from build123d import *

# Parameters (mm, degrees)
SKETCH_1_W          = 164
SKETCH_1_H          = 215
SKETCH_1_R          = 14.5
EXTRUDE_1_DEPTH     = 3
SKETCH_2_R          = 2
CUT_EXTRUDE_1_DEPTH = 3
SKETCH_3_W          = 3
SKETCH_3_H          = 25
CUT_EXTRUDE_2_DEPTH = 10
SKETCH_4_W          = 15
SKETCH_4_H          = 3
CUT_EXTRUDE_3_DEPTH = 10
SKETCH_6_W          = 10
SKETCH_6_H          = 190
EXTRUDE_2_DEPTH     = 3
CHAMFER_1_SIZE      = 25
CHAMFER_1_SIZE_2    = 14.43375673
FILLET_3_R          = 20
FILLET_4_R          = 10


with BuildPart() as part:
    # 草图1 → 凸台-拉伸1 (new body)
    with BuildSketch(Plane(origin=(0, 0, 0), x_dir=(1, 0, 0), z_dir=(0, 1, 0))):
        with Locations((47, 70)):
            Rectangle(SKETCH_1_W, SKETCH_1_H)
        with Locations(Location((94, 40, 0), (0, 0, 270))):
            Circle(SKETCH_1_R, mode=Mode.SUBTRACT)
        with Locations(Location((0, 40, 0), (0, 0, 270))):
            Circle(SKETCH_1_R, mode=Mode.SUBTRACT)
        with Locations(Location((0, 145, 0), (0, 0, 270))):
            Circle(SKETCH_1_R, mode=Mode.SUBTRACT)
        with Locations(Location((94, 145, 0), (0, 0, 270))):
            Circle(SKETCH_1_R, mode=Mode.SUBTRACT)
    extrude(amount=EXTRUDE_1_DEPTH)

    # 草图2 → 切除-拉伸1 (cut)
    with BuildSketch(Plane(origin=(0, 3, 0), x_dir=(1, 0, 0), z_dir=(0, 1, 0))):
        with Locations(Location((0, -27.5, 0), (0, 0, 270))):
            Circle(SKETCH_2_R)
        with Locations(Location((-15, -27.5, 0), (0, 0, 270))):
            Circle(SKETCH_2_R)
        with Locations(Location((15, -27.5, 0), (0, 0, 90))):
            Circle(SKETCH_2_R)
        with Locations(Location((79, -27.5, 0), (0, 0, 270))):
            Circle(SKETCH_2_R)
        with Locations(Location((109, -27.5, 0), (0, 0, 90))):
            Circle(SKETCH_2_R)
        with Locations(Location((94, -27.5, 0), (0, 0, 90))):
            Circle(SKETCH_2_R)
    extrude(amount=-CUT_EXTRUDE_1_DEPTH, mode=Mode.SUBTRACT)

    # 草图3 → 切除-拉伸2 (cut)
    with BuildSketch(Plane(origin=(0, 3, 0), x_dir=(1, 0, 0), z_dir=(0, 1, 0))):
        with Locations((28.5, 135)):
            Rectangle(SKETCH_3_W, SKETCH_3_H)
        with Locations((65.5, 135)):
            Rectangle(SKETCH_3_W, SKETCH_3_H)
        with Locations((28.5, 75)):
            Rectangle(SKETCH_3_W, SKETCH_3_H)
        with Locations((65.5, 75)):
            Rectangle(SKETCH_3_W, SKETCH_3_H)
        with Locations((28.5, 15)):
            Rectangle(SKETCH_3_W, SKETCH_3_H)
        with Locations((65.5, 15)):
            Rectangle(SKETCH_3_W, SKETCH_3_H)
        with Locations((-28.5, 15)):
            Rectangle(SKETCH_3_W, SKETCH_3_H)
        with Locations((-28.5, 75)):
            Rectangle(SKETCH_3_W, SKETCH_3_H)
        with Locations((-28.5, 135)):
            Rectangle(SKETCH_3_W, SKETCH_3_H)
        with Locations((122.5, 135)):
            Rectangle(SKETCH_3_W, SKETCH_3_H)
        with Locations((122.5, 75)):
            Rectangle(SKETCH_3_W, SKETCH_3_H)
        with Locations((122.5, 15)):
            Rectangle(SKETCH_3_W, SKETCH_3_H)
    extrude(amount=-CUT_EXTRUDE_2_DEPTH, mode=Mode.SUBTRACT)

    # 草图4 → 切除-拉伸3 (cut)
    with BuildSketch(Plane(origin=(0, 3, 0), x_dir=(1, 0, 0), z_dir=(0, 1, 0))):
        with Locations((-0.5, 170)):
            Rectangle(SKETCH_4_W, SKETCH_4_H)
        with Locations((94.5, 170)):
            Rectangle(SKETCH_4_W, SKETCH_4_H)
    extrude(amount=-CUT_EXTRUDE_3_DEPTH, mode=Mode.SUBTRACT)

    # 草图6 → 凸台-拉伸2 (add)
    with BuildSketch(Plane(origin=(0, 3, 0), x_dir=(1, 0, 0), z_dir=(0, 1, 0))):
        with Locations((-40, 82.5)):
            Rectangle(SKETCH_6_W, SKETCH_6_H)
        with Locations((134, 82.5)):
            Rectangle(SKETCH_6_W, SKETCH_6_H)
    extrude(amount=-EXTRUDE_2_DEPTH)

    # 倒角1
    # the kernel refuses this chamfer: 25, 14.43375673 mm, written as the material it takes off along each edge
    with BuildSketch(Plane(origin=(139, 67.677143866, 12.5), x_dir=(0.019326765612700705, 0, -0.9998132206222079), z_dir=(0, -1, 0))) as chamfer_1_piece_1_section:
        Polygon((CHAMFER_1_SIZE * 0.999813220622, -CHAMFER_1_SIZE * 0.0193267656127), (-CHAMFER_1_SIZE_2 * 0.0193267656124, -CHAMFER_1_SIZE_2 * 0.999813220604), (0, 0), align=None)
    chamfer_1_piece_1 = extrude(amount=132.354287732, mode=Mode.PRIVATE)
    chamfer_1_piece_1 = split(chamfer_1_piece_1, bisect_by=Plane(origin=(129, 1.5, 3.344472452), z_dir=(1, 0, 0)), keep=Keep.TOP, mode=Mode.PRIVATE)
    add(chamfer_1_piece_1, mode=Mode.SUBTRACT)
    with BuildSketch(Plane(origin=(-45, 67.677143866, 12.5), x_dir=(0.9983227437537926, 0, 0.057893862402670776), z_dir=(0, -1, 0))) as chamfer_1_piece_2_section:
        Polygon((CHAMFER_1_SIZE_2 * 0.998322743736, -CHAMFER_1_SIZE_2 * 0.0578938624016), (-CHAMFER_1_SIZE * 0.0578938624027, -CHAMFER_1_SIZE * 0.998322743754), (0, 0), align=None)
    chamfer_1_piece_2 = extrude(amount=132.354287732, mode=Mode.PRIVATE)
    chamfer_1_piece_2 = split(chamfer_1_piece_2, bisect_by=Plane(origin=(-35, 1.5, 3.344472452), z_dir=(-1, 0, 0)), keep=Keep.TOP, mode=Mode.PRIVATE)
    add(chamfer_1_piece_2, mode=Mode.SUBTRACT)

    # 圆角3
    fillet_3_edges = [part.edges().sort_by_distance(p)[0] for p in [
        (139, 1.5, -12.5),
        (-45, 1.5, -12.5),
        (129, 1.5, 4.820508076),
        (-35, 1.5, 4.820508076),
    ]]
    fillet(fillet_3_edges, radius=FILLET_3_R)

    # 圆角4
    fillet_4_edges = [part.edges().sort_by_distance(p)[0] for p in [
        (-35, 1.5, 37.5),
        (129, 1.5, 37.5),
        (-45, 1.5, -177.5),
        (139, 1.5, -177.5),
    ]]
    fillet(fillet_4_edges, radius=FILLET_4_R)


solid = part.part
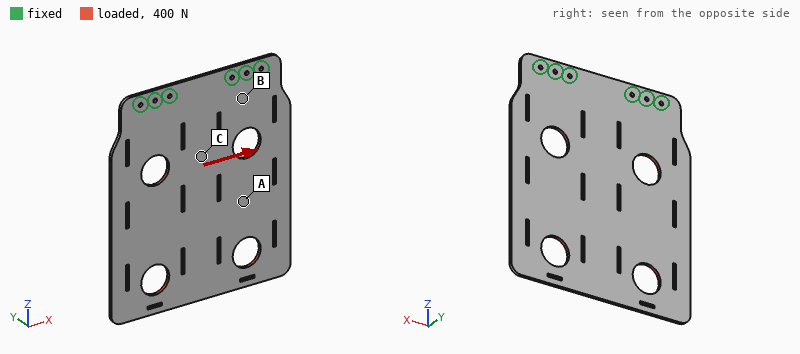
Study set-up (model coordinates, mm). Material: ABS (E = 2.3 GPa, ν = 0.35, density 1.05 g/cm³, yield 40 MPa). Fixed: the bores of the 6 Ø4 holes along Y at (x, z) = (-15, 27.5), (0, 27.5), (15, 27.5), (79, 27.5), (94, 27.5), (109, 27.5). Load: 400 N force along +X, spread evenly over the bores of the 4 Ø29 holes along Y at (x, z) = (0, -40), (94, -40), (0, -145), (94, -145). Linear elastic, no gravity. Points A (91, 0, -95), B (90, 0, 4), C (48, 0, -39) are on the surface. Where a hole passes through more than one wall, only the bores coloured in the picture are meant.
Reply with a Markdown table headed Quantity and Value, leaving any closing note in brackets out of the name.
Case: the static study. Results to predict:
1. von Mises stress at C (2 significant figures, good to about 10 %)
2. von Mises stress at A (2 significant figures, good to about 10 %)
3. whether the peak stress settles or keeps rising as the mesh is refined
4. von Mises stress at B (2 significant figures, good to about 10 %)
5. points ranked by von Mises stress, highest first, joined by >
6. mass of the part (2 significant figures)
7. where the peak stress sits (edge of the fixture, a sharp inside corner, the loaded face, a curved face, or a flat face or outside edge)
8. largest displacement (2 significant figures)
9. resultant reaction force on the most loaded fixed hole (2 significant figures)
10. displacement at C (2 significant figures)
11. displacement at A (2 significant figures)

| Quantity | Value |
|---|---|
| von Mises stress at C | 1.8 MPa |
| von Mises stress at A | 0.80 MPa |
| whether the peak stress settles or keeps rising as the mesh is refined | keeps rising |
| von Mises stress at B | 2.9 MPa |
| points ranked by von Mises stress, highest first, joined by > | B > C > A |
| mass of the part | 110 g |
| where the peak stress sits | edge of the fixture |
| largest displacement | 0.55 mm |
| resultant reaction force on the most loaded fixed hole | 300 N |
| displacement at C | 0.16 mm |
| displacement at A | 0.33 mm |
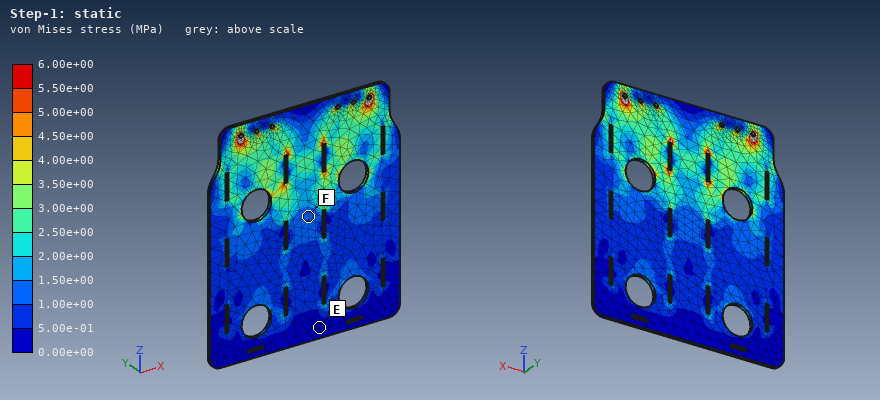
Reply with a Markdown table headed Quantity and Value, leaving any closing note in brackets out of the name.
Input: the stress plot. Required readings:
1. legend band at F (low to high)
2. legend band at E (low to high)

| Quantity | Value |
|---|---|
| legend band at F | 1.00e+00 to 1.50e+00 MPa |
| legend band at E | 0.00e+00 to 5.00e-01 MPa |
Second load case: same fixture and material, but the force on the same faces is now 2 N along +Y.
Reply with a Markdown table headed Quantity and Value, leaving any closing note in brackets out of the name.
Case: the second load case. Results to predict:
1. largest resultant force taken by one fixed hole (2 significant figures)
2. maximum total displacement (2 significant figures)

| Quantity | Value |
|---|---|
| largest resultant force taken by one fixed hole | 1.1 N |
| maximum total displacement | 3.2 mm |
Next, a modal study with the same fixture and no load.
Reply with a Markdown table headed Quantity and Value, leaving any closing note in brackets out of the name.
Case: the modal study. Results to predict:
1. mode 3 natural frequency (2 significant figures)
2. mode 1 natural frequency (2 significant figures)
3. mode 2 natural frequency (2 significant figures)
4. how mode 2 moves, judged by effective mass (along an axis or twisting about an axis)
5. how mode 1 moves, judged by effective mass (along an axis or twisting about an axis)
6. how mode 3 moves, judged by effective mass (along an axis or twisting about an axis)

| Quantity | Value |
|---|---|
| mode 3 natural frequency | 100 Hz |
| mode 1 natural frequency | 17 Hz |
| mode 2 natural frequency | 44 Hz |
| how mode 2 moves, judged by effective mass | twisting about Z |
| how mode 1 moves, judged by effective mass | along Y |
| how mode 3 moves, judged by effective mass | along Y |
